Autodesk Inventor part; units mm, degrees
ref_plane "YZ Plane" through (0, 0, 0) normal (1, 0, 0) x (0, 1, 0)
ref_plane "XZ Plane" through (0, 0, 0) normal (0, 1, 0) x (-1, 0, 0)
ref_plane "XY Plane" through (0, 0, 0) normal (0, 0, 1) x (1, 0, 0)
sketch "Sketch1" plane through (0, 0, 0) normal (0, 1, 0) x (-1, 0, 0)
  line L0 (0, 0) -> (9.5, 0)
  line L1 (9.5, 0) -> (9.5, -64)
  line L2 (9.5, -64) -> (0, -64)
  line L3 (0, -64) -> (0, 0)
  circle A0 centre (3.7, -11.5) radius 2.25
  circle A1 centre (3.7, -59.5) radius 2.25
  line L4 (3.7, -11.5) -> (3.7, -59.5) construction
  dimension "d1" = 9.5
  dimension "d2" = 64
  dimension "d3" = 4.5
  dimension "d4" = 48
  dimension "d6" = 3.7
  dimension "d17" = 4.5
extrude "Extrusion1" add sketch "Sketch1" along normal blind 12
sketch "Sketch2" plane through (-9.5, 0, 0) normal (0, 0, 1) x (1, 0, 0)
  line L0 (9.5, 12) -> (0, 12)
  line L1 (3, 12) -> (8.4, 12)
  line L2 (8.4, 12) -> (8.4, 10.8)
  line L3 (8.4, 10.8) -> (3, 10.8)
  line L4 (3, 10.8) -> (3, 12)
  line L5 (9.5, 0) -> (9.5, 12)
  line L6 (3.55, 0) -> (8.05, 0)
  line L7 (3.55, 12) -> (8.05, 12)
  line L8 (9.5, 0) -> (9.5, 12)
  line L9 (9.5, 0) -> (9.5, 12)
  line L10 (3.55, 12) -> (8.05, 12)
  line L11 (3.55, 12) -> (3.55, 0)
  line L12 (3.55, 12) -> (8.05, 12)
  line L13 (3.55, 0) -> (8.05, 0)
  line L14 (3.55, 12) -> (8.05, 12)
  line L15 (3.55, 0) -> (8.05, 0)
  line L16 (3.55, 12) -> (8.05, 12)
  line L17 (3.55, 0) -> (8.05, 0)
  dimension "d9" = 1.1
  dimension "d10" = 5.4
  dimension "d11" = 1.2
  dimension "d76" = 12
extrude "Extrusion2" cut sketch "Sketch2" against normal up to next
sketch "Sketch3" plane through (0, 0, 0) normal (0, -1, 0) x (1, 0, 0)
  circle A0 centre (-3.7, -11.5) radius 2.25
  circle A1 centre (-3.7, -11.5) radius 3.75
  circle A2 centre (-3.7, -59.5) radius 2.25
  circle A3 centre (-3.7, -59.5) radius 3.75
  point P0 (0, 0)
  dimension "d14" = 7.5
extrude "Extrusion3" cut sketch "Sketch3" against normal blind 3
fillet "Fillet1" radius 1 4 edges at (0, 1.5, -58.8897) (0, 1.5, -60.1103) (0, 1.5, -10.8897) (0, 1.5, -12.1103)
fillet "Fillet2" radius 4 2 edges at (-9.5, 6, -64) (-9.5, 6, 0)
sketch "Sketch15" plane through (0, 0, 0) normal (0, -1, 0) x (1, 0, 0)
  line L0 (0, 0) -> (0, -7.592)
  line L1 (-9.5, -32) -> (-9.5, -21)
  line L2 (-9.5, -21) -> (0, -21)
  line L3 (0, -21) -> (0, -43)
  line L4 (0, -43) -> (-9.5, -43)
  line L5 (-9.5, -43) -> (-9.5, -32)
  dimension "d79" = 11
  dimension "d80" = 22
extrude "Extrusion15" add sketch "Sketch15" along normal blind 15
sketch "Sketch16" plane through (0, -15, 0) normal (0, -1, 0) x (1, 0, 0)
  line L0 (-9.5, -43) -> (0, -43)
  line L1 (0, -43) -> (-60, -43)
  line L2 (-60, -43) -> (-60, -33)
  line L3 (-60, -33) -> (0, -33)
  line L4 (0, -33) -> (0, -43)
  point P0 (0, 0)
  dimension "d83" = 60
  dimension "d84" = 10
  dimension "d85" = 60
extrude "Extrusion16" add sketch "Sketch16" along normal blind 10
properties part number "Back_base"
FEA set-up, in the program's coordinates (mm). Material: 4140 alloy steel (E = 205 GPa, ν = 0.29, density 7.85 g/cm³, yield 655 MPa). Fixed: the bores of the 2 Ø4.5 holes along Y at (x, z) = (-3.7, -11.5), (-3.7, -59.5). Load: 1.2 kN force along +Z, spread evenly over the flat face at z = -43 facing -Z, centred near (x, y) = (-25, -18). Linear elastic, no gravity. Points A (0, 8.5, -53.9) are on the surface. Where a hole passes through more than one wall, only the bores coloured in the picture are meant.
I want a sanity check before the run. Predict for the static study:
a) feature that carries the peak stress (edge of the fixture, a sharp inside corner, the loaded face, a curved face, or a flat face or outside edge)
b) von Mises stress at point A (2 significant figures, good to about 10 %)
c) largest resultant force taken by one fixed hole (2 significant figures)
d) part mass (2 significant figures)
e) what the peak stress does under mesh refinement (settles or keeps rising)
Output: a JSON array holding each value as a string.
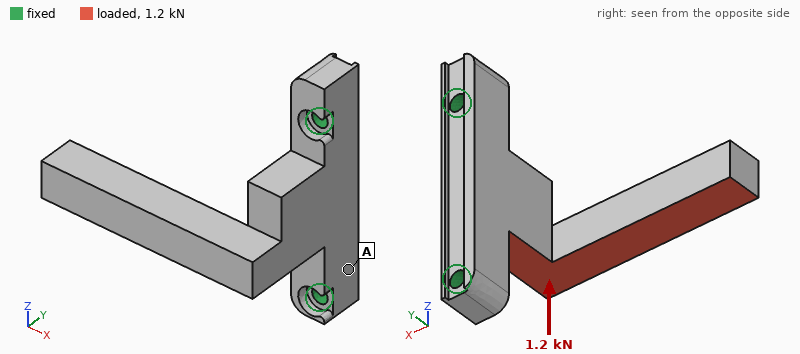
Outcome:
["a sharp inside corner", "34 MPa", "1.2 kN", "120 g", "keeps rising"]
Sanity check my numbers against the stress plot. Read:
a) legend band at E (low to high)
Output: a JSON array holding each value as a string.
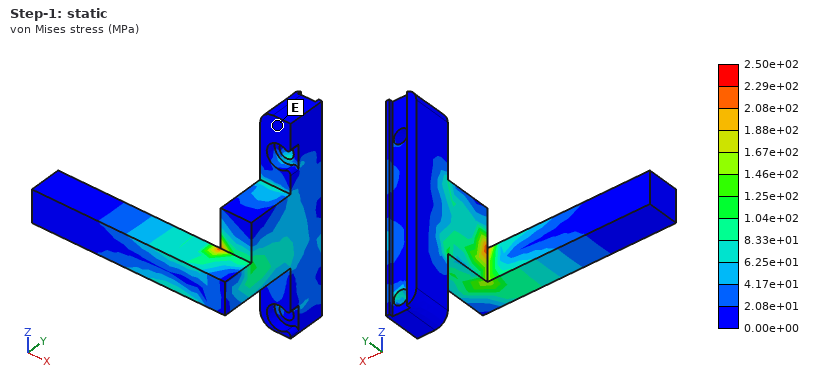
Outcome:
["0.00e+00 to 2.08e+01 MPa"]
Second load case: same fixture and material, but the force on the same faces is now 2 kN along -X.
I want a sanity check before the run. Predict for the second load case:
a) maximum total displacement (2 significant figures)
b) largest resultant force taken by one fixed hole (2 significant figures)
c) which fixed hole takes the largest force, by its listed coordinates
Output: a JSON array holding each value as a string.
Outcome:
["0.36 mm", "1.4 kN", "(-3.7, -59.5)"]
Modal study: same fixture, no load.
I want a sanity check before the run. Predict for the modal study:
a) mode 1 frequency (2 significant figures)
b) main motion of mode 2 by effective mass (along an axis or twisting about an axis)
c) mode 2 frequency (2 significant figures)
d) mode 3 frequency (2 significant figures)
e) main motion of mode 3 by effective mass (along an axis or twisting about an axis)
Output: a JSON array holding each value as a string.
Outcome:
["1400 Hz", "along Z", "1800 Hz", "4000 Hz", "along X"]
